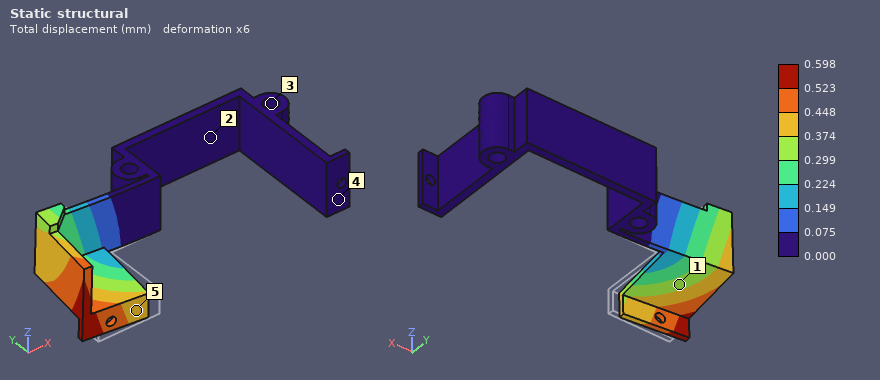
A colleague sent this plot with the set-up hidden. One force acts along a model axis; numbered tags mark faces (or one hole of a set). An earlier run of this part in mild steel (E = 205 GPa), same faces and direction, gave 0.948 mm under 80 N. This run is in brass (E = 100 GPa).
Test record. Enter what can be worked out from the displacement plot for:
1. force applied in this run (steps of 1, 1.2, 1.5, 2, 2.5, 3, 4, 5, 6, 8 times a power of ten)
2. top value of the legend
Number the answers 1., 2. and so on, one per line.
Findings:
1. 25 N
2. 0.598 mm
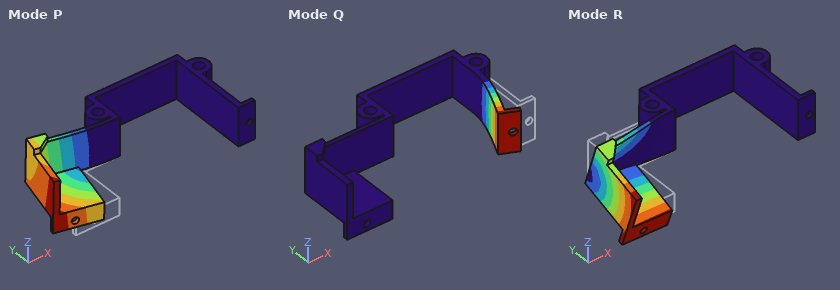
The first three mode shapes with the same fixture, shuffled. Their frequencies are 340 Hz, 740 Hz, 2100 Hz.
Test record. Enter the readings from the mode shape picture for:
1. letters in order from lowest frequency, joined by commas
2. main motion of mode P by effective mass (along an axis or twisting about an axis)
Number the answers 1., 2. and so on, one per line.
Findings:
1. P, R, Q
2. along Y
